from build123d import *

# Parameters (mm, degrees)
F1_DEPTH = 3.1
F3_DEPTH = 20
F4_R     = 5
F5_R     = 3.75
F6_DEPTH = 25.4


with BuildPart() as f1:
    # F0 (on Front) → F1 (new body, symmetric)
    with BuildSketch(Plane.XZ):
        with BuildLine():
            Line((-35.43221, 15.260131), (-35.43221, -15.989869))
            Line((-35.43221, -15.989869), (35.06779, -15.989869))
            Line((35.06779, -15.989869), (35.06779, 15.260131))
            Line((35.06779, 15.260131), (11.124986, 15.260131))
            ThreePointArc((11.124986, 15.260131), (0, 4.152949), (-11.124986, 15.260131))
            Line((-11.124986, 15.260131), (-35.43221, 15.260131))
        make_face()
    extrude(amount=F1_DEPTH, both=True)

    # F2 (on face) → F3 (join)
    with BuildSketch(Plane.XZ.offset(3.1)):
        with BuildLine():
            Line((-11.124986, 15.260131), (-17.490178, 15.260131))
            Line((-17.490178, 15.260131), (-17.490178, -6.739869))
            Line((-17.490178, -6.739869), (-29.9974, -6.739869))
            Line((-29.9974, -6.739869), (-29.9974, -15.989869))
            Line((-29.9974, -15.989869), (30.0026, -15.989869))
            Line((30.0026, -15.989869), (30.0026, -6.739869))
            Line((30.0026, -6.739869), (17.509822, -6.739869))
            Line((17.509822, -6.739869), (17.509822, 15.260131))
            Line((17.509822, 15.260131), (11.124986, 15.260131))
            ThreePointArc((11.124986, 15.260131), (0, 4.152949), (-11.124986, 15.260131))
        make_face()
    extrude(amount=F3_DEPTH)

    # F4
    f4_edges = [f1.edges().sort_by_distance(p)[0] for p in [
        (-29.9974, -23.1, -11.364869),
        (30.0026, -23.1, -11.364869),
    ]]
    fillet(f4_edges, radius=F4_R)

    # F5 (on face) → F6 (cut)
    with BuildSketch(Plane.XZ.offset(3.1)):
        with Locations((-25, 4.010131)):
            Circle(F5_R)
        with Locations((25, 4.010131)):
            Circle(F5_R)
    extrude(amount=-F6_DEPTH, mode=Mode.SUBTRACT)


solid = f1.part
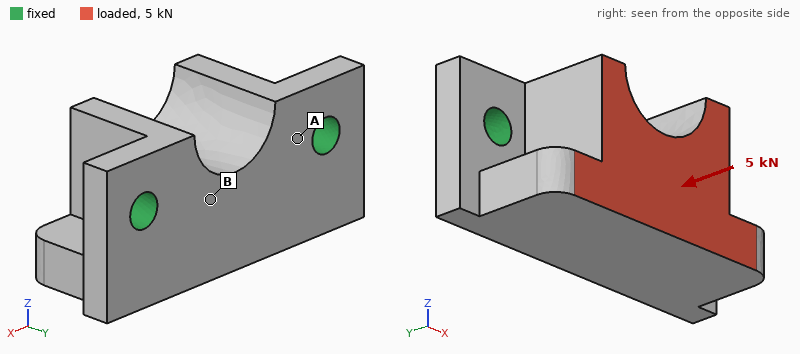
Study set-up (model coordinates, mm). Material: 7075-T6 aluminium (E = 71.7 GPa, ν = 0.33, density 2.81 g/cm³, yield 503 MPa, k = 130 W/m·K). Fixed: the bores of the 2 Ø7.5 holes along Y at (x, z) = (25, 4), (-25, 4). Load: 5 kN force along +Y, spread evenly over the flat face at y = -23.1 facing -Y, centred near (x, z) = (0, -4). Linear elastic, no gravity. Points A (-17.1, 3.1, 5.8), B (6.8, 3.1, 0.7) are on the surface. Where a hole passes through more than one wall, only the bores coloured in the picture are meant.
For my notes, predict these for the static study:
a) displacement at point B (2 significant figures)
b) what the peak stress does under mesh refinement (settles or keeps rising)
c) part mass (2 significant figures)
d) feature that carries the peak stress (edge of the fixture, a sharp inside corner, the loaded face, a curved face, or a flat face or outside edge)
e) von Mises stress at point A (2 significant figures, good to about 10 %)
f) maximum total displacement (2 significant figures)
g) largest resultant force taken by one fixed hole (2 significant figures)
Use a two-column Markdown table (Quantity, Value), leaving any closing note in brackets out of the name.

| Quantity | Value |
|---|---|
| displacement at point B | 14 µm |
| what the peak stress does under mesh refinement | keeps rising |
| part mass | 97 g |
| feature that carries the peak stress | edge of the fixture |
| von Mises stress at point A | 23 MPa |
| maximum total displacement | 54 µm |
| largest resultant force taken by one fixed hole | 2.6 kN |
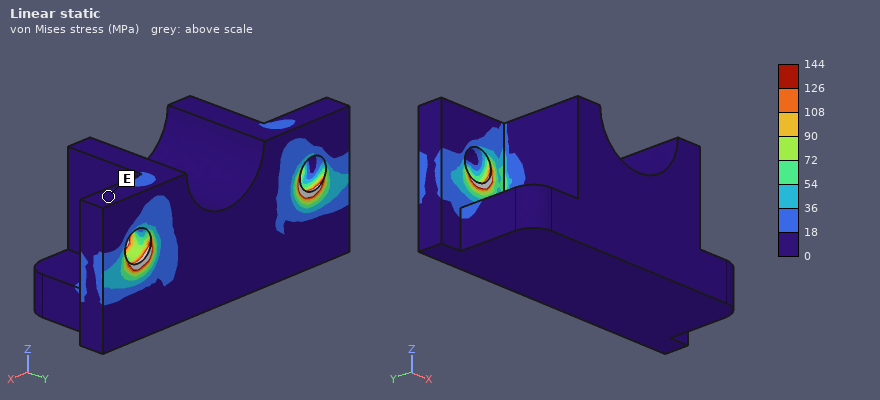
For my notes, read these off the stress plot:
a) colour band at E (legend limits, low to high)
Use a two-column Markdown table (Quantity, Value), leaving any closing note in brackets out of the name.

| Quantity | Value |
|---|---|
| colour band at E | 0 to 18 MPa |
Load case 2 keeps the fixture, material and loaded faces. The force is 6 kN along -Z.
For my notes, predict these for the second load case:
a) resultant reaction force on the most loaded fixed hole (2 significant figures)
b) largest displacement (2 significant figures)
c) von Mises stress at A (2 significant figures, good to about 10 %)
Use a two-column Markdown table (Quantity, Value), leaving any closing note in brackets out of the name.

| Quantity | Value |
|---|---|
| resultant reaction force on the most loaded fixed hole | 3.4 kN |
| largest displacement | 0.22 mm |
| von Mises stress at A | 98 MPa |
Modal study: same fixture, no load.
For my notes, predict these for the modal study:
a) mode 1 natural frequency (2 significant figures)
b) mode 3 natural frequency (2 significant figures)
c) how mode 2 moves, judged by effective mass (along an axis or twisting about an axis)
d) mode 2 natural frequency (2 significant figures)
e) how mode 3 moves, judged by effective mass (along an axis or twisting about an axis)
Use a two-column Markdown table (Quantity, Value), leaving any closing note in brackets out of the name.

| Quantity | Value |
|---|---|
| mode 1 natural frequency | 4600 Hz |
| mode 3 natural frequency | 13 kHz |
| how mode 2 moves, judged by effective mass | along X |
| mode 2 natural frequency | 12 kHz |
| how mode 3 moves, judged by effective mass | along Y |
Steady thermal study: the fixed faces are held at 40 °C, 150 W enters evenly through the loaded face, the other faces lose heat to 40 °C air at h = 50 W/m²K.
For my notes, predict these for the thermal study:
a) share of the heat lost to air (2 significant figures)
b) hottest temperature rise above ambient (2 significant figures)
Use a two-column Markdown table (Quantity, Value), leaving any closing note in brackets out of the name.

| Quantity | Value |
|---|---|
| share of the heat lost to air | 7.8 % |
| hottest temperature rise above ambient | 54 K |
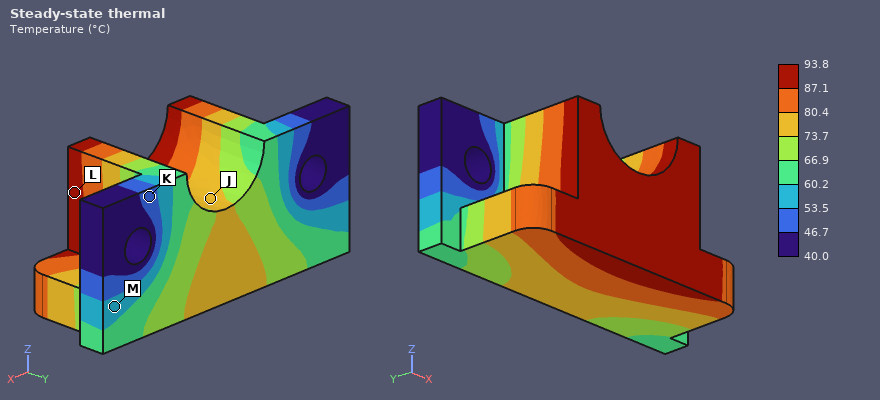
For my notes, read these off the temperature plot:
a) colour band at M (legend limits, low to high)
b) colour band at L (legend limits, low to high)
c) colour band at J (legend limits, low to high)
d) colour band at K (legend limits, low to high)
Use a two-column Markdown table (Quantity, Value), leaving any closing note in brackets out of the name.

| Quantity | Value |
|---|---|
| colour band at M | 53.5 to 60.2 °C |
| colour band at L | 87.1 to 93.8 °C |
| colour band at J | 73.7 to 80.4 °C |
| colour band at K | 46.7 to 53.5 °C |
